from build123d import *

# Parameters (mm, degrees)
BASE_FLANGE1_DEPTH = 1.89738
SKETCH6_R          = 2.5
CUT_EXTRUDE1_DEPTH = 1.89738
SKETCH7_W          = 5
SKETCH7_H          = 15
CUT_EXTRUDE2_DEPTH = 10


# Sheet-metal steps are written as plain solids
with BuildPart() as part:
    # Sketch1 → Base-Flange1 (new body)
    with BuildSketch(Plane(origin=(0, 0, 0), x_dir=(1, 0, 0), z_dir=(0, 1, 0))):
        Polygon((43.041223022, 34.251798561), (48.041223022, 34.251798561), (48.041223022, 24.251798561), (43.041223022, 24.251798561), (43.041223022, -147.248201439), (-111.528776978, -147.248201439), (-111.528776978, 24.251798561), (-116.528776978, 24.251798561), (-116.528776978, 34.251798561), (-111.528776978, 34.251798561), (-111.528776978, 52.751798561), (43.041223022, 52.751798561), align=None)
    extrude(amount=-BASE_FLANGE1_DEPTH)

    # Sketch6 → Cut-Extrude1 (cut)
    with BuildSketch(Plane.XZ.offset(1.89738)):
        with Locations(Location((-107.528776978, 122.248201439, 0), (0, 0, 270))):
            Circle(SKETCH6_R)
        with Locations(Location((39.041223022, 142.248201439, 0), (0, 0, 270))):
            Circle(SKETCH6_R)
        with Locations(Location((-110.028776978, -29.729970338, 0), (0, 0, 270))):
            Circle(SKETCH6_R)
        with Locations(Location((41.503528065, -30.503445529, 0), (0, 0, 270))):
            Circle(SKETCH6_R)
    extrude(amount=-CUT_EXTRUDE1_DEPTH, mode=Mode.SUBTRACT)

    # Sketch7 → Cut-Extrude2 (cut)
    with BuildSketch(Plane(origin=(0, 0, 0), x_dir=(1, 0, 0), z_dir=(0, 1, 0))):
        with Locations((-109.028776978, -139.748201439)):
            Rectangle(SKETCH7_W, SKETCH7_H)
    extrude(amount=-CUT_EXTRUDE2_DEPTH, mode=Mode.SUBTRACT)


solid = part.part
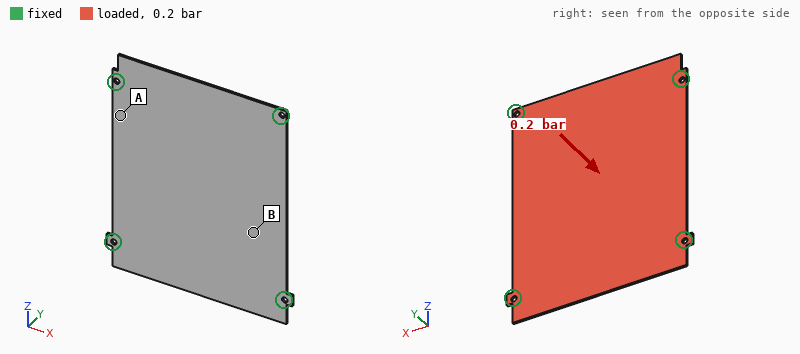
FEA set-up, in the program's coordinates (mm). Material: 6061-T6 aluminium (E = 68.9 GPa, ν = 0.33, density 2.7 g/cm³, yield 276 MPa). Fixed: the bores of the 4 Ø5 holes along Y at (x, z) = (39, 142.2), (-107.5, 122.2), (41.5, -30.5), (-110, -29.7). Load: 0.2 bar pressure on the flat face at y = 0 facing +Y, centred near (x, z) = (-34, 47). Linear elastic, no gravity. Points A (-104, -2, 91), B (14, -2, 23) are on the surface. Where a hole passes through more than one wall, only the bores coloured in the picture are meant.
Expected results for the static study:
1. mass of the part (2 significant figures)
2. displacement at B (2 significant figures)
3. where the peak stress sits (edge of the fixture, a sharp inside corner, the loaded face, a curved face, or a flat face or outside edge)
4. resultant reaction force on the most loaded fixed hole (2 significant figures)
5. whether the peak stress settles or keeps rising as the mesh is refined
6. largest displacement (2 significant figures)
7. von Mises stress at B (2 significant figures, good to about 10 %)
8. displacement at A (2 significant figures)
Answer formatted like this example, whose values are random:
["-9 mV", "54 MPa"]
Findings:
["160 g", "1.9 mm", "edge of the fixture", "170 N", "keeps rising", "2.4 mm", "42 MPa", "0.60 mm"]
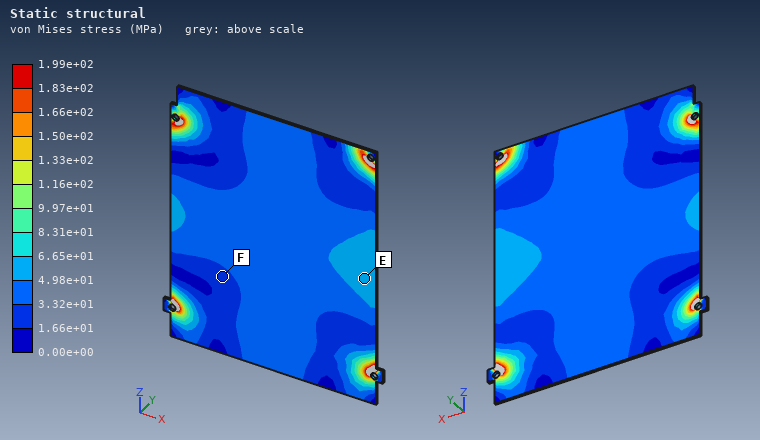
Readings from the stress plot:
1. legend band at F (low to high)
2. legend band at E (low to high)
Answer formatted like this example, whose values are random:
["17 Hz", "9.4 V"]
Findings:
["1.66e+01 to 3.32e+01 MPa", "4.98e+01 to 6.65e+01 MPa"]
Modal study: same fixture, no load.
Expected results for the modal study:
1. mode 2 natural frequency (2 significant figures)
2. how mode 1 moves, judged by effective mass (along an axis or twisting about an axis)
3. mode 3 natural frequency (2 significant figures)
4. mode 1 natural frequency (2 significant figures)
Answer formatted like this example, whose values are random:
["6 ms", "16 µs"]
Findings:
["410 Hz", "along Y", "450 Hz", "240 Hz"]
